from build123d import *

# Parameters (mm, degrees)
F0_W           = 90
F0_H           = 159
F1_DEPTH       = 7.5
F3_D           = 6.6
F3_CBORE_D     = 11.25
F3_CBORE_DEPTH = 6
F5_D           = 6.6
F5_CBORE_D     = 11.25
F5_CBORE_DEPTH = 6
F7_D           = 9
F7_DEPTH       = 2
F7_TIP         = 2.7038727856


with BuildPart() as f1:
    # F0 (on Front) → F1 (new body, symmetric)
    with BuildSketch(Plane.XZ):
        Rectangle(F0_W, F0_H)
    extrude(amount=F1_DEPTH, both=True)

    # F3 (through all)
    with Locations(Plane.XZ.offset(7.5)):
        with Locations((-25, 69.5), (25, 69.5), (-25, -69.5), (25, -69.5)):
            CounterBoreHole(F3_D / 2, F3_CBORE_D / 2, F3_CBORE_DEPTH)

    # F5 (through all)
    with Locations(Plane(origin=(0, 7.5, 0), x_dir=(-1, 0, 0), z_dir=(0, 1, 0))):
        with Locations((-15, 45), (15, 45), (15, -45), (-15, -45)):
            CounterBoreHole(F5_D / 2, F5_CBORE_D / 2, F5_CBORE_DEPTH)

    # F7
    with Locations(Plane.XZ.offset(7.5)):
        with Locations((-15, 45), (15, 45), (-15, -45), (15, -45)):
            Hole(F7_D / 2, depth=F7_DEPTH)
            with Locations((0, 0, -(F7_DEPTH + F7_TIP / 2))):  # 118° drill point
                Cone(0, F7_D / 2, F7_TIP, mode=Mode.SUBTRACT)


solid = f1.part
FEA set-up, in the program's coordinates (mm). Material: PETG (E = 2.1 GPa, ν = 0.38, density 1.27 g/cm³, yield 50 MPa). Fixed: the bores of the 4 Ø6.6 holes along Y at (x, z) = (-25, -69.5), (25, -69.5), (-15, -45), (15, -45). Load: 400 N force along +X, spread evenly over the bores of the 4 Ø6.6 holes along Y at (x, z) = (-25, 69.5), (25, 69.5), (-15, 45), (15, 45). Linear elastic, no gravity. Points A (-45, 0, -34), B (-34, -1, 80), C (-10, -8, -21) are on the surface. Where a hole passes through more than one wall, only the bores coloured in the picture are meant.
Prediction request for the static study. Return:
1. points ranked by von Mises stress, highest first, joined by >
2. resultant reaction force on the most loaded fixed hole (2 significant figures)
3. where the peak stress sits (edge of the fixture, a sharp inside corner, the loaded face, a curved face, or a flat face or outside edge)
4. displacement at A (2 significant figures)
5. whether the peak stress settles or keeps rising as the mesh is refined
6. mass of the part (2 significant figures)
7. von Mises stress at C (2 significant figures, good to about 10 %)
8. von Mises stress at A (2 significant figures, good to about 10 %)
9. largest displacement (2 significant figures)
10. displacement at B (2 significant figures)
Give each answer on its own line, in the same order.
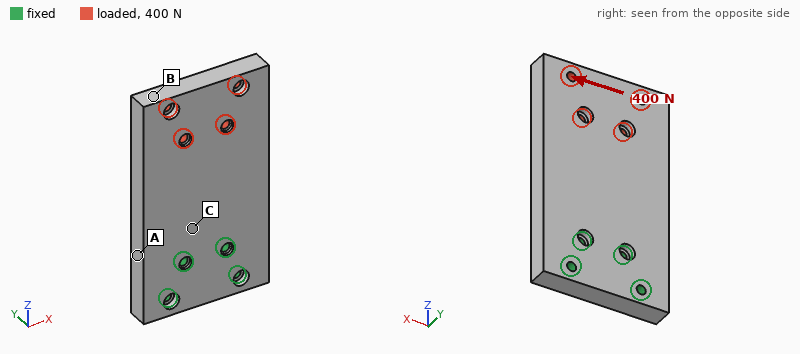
A > C > B
550 N
edge of the fixture
0.059 mm
keeps rising
260 g
0.92 MPa
1.7 MPa
0.28 mm
0.27 mm
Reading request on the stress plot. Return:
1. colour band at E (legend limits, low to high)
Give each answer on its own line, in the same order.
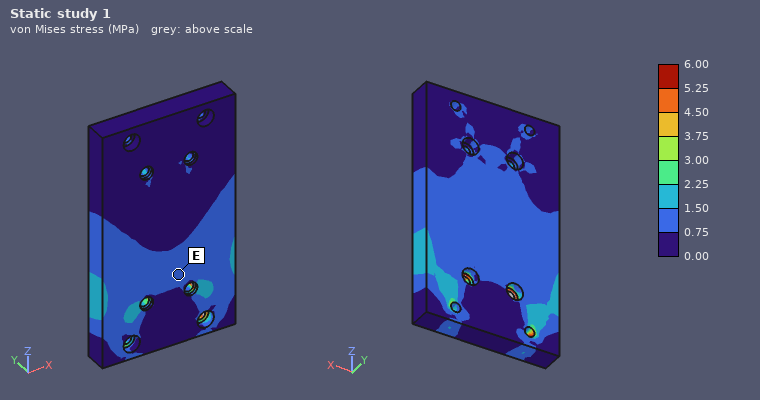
0.75 to 1.50 MPa
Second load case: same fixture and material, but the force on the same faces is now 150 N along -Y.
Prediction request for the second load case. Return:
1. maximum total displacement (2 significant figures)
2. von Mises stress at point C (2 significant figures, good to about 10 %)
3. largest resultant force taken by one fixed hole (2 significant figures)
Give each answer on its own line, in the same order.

1.8 mm
3.2 MPa
310 N
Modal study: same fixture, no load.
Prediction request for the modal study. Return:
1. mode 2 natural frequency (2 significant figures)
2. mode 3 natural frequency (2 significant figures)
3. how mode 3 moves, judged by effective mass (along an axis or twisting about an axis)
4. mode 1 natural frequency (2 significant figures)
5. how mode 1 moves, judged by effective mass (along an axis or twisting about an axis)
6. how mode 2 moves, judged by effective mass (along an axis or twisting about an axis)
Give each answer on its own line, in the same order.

490 Hz
680 Hz
along X
180 Hz
along Y
twisting about Z
